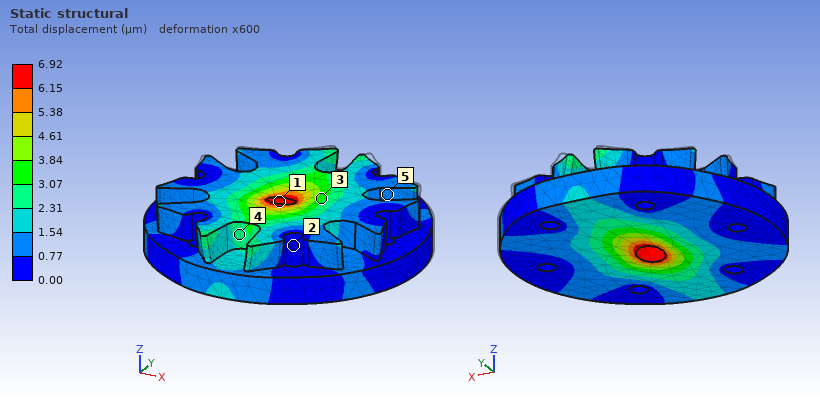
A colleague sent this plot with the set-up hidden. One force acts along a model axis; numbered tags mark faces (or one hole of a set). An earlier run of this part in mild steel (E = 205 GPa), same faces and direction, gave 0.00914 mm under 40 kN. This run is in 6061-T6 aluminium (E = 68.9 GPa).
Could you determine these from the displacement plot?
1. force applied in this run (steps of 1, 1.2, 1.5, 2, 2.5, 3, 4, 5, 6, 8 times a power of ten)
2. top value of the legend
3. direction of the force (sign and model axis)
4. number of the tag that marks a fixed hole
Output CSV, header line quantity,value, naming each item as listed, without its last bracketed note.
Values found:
quantity,value
force applied in this run,10 kN
top value of the legend,6.92 µm
direction of the force,-Y
number of the tag that marks a fixed hole,2
